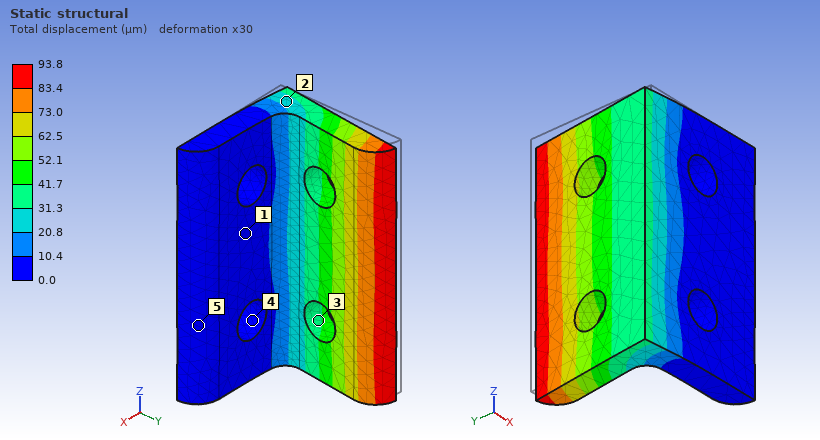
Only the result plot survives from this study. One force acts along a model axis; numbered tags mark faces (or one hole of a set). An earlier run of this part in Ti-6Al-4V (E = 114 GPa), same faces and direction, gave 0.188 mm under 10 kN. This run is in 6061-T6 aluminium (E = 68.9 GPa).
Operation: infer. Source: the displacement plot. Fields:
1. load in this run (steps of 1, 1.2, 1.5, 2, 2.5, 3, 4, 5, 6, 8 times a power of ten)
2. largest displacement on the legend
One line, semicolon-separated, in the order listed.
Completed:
3 kN; 93.8 µm
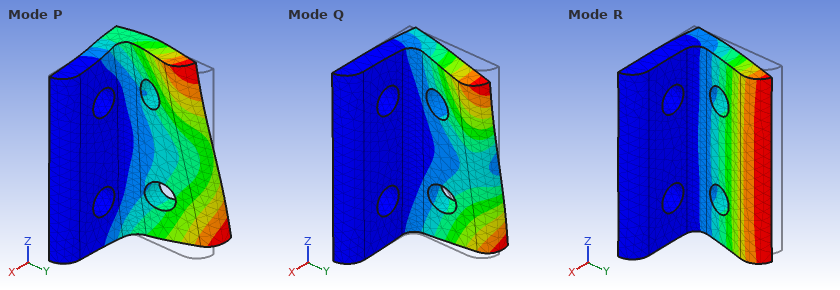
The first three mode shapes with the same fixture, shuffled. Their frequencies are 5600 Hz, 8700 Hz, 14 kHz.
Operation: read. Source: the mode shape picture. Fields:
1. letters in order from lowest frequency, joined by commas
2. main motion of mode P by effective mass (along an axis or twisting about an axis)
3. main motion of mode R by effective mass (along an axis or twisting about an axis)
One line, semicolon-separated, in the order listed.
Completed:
R, Q, P; along Z; along X
